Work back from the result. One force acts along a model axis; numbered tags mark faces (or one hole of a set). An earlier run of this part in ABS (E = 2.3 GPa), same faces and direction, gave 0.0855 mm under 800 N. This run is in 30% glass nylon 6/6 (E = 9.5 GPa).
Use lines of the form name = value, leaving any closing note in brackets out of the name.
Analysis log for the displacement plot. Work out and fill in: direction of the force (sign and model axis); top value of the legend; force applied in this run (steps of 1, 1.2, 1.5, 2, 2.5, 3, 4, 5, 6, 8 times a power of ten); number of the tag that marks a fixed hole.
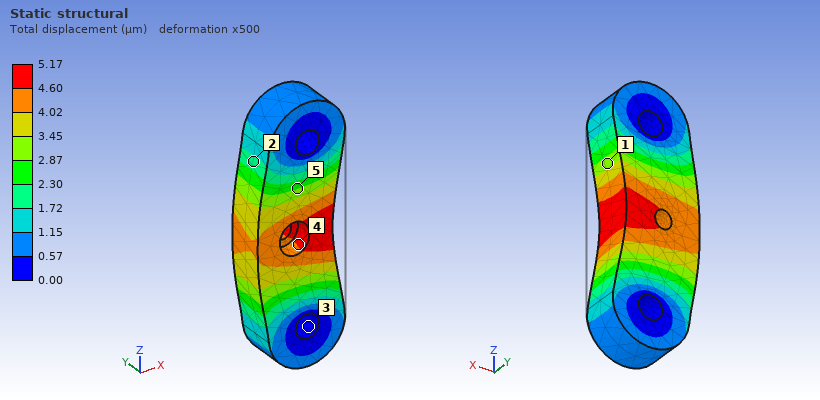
direction of the force = -X
top value of the legend = 5.17 µm
force applied in this run = 200 N
number of the tag that marks a fixed hole = 3
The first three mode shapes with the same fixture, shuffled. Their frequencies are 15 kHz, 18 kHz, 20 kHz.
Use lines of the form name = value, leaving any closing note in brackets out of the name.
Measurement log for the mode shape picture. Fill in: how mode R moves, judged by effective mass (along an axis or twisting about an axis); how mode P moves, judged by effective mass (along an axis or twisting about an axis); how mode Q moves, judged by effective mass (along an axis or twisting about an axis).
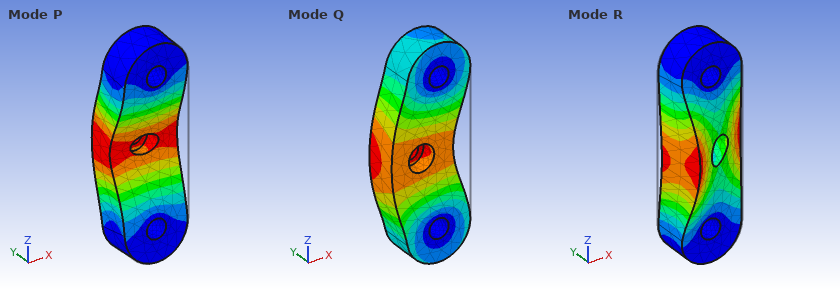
how mode R moves, judged by effective mass = twisting about Z
how mode P moves, judged by effective mass = along Y
how mode Q moves, judged by effective mass = along X
